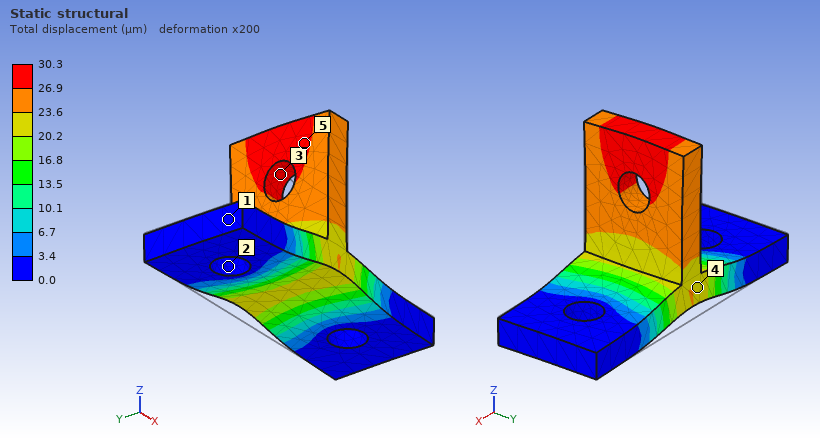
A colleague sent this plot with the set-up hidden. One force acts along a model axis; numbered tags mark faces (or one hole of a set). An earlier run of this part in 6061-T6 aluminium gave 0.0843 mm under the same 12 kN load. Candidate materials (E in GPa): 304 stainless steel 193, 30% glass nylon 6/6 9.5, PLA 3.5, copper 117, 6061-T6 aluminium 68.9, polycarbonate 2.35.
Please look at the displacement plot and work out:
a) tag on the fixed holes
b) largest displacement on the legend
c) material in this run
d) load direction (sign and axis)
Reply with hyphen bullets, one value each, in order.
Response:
- 2
- 30.3 µm
- 304 stainless steel
- +Z
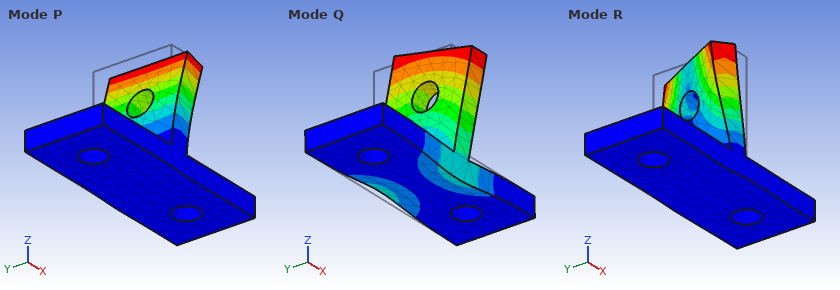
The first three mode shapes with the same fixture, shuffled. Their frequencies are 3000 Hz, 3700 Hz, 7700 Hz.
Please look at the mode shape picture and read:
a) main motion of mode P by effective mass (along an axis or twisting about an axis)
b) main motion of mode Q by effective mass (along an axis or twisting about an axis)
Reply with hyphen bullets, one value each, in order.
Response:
- along X
- along Y
